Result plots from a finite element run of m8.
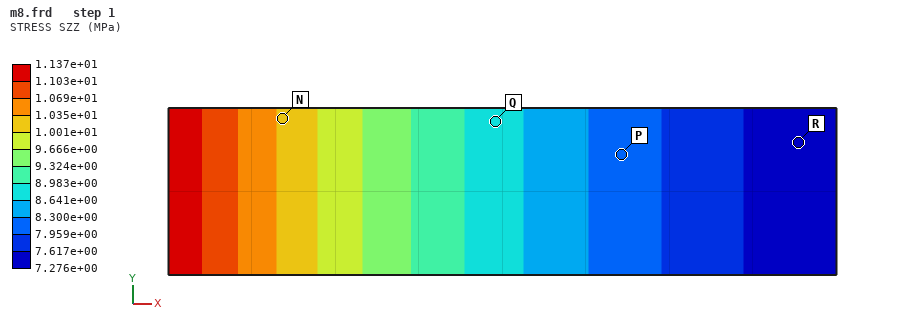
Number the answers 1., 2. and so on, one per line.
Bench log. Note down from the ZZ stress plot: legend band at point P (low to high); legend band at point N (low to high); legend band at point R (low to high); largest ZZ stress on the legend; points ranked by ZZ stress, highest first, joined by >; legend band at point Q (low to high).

1. 7.959e+00 to 8.300e+00 MPa
2. 1.001e+01 to 1.035e+01 MPa
3. 7.276e+00 to 7.617e+00 MPa
4. 1.137e+01 MPa
5. N > Q > P > R
6. 8.641e+00 to 8.983e+00 MPa
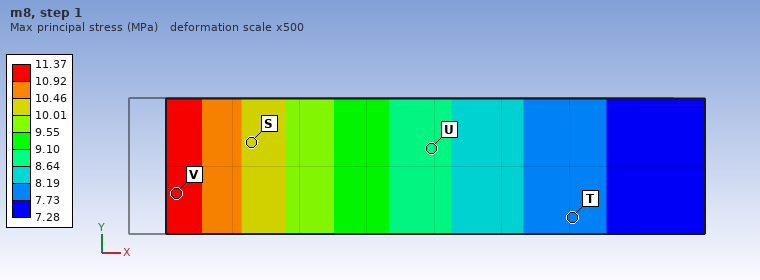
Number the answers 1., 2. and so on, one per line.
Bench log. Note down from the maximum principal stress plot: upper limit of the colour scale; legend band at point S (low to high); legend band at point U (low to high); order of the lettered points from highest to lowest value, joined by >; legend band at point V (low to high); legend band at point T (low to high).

1. 11.37 MPa
2. 10.01 to 10.46 MPa
3. 8.64 to 9.10 MPa
4. V > S > U > T
5. 10.92 to 11.37 MPa
6. 7.73 to 8.19 MPa
